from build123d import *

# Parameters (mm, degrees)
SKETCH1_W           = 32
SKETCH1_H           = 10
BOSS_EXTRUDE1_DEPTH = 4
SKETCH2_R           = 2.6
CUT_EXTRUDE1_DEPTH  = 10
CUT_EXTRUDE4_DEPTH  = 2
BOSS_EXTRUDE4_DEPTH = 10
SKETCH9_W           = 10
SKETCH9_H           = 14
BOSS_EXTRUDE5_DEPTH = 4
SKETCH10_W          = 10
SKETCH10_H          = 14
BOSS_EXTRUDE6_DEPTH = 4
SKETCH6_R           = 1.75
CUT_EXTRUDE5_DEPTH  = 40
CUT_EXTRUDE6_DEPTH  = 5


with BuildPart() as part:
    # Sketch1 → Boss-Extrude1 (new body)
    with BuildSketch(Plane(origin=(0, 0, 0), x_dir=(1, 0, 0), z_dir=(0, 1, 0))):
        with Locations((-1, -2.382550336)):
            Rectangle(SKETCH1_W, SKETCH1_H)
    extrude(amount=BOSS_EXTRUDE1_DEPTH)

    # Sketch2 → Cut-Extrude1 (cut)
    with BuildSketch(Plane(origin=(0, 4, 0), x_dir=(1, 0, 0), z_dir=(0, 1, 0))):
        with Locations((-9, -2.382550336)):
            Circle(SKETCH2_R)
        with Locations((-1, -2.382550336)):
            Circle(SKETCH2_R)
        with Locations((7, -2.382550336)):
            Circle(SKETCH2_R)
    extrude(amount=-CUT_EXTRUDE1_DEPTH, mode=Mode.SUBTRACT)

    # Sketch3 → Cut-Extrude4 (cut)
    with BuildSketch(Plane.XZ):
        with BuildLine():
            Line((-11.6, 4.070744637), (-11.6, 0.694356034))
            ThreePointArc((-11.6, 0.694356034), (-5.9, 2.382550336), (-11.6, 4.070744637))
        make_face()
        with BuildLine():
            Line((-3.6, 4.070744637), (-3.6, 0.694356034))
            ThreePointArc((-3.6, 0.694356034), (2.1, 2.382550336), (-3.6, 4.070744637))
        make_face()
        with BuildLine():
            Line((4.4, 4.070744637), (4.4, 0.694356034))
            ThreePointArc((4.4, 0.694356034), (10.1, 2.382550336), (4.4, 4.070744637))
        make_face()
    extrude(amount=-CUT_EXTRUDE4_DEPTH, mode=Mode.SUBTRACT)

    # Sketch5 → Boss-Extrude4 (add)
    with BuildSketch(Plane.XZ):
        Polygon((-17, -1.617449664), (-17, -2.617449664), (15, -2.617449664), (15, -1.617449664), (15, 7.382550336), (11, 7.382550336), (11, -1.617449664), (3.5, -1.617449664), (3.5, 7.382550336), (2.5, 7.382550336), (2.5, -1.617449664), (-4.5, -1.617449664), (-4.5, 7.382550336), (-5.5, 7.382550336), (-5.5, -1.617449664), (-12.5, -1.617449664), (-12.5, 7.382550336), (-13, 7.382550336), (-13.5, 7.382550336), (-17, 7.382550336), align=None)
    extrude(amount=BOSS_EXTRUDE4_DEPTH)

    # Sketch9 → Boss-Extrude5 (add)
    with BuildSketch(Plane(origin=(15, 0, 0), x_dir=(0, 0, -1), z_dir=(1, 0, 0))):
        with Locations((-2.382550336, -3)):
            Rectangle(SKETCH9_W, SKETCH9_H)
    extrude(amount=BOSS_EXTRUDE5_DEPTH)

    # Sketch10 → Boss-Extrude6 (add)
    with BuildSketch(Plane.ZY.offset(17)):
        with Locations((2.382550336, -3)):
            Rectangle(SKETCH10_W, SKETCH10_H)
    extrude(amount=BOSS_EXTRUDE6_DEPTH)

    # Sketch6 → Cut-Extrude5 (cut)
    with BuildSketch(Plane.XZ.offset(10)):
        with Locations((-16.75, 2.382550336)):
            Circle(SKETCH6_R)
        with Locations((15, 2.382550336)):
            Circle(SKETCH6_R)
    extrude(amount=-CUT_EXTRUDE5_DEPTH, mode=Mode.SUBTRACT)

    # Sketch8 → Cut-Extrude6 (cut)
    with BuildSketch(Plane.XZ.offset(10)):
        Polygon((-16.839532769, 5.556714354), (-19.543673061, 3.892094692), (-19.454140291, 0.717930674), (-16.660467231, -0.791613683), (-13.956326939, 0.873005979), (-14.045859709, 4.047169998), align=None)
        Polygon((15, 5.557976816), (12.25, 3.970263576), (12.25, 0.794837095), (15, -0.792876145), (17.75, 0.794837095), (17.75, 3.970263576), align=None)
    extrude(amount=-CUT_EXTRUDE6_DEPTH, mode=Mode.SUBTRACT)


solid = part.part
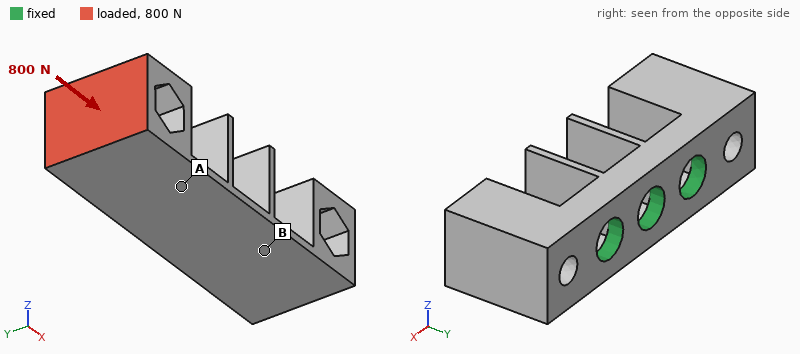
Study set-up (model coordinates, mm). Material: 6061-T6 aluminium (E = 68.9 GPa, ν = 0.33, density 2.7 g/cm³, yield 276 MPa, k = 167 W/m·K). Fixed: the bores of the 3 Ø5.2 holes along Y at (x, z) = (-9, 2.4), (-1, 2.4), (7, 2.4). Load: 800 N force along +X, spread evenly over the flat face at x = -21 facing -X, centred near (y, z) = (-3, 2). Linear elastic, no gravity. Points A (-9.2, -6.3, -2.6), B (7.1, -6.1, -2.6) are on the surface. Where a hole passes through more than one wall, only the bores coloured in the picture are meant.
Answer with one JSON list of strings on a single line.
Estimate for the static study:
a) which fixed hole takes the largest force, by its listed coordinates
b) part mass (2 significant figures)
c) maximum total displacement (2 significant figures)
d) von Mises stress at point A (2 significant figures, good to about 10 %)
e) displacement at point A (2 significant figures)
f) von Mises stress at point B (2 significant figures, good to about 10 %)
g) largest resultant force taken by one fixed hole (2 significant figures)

["(-9, 2.4)", "7.9 g", "38 µm", "37 MPa", "9.9 µm", "10 MPa", "500 N"]
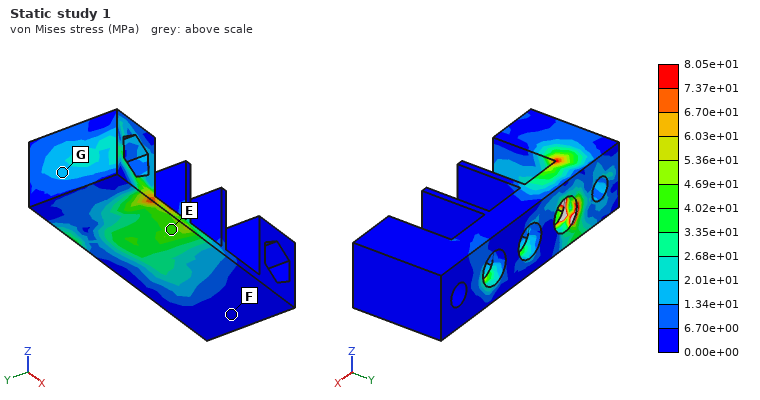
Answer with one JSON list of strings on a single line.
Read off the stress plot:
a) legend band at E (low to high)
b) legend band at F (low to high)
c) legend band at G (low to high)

["4.02e+01 to 4.69e+01 MPa", "0.00e+00 to 6.70e+00 MPa", "1.34e+01 to 2.01e+01 MPa"]
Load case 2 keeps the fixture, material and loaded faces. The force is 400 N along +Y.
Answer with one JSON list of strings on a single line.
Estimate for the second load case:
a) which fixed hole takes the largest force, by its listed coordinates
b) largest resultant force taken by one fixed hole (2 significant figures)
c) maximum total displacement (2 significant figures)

["(-9, 2.4)", "670 N", "35 µm"]
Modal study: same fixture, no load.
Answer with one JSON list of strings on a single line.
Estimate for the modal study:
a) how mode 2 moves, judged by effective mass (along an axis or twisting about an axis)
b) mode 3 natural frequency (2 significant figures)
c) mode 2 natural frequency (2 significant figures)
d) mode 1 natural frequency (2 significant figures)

["along Z", "15 kHz", "14 kHz", "12 kHz"]
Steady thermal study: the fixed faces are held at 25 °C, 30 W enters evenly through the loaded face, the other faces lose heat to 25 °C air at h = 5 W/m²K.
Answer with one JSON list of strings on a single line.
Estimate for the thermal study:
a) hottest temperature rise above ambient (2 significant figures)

["41 K"]
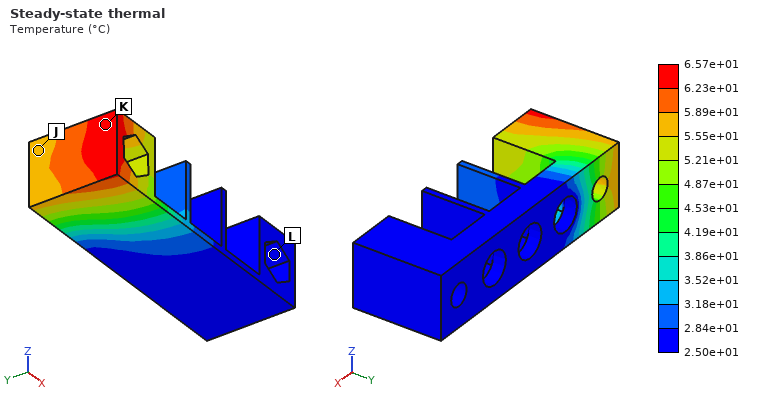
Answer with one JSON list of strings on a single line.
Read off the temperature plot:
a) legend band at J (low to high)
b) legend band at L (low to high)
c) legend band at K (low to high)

["5.55e+01 to 5.89e+01 °C", "2.50e+01 to 2.84e+01 °C", "6.23e+01 to 6.57e+01 °C"]
